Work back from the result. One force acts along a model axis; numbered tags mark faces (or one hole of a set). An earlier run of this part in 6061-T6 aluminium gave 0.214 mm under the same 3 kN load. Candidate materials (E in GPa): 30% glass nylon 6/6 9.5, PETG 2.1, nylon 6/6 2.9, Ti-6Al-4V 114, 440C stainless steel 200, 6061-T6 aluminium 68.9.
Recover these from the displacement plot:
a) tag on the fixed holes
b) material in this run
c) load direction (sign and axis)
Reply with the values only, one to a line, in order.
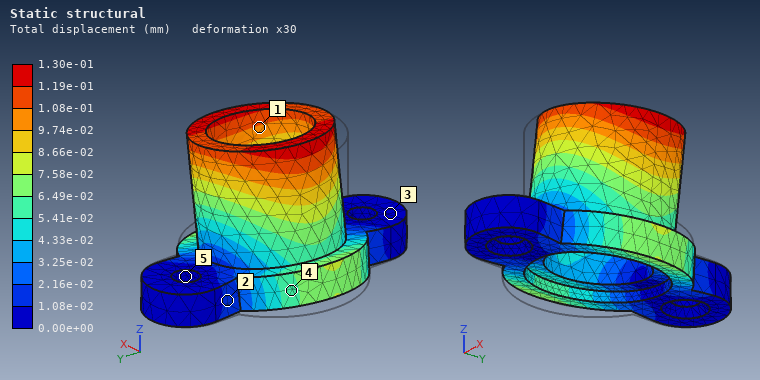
5
Ti-6Al-4V
+X
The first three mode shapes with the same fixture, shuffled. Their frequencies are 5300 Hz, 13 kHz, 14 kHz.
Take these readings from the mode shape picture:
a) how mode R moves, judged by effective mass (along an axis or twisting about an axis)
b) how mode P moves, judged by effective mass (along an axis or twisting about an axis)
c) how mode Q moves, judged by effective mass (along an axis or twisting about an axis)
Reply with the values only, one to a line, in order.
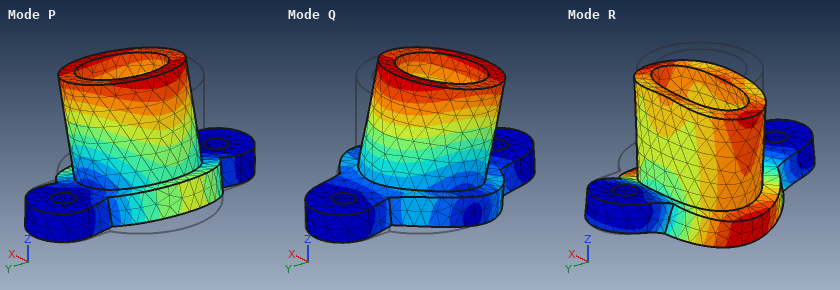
along Z
along X
along Y
